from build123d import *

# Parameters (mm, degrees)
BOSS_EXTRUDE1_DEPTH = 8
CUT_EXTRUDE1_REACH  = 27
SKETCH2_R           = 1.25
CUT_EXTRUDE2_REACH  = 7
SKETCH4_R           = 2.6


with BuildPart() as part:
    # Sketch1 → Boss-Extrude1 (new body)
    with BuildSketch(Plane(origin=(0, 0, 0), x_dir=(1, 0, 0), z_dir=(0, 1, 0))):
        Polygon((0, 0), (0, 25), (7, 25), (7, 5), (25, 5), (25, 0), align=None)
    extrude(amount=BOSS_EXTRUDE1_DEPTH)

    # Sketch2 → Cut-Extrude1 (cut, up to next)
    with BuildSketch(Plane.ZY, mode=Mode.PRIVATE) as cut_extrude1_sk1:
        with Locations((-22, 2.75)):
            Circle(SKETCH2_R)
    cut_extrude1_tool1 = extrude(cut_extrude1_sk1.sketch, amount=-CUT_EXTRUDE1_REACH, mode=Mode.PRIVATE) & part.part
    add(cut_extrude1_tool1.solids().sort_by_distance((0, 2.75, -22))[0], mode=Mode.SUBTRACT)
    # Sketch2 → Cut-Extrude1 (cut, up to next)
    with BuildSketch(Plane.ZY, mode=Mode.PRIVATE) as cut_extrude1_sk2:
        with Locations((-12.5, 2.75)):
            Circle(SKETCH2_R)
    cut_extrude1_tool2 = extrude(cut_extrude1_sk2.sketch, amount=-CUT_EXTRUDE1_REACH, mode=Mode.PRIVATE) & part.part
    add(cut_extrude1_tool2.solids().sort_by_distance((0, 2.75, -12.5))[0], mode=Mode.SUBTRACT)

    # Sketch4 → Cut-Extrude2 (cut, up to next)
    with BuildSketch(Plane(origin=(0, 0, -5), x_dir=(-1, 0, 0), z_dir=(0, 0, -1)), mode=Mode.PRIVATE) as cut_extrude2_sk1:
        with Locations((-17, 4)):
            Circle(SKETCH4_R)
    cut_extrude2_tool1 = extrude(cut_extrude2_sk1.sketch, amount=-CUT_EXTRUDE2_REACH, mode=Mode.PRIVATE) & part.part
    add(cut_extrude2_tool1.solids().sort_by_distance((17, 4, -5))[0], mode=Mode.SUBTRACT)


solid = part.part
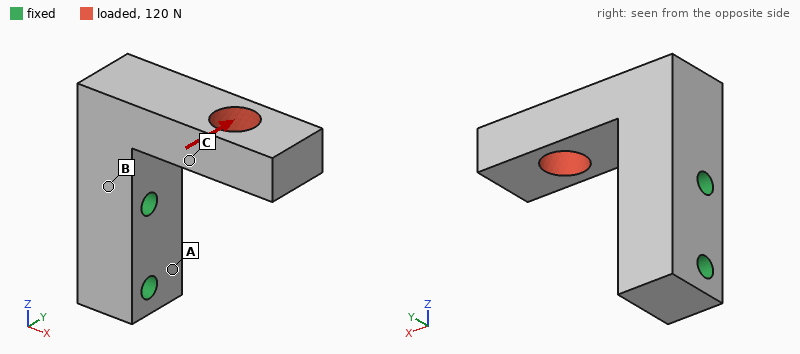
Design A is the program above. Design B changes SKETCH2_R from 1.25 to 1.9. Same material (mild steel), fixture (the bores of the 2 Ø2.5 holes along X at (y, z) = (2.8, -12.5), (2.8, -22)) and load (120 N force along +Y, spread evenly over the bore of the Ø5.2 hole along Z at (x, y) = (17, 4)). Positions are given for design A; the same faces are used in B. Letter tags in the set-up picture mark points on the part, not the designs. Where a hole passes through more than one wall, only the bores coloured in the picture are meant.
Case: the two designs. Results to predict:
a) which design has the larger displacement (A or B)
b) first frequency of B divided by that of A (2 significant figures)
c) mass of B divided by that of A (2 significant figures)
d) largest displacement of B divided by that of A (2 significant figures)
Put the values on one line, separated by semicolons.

A; 1.0; 0.95; 0.91
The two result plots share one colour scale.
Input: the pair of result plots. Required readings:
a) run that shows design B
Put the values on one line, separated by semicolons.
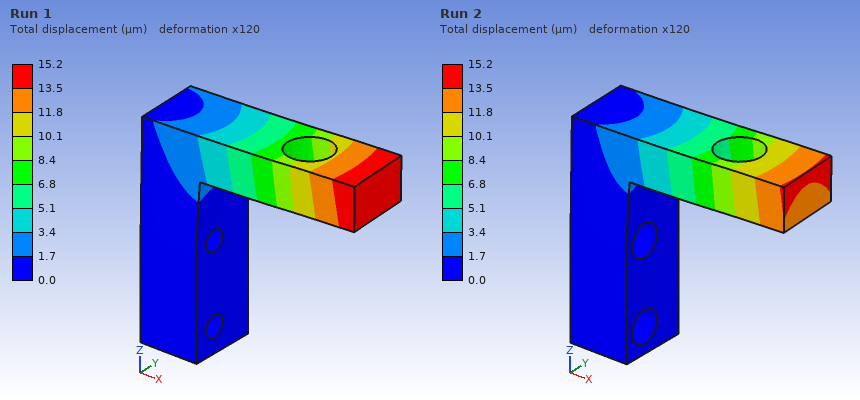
Run 2
